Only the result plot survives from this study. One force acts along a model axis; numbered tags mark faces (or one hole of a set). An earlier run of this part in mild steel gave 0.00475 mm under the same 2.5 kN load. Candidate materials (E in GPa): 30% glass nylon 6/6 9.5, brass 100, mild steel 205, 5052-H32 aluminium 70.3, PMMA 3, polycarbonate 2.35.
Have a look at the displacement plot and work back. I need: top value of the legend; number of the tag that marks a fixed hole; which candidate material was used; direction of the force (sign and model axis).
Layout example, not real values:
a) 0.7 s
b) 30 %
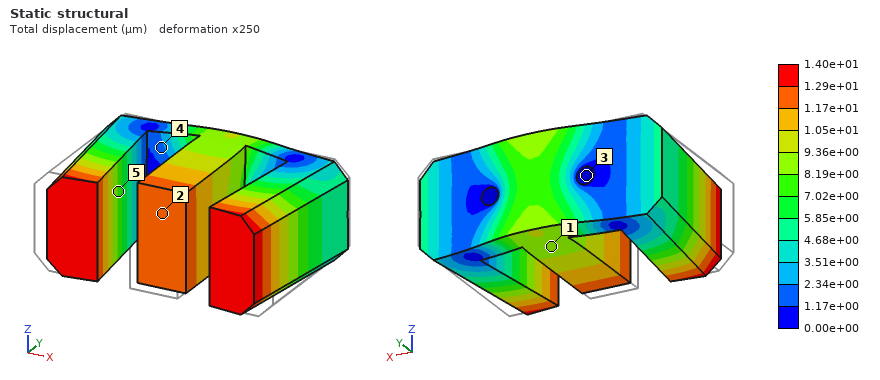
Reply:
a) 1.40e+01 µm
b) 3
c) 5052-H32 aluminium
d) +Y
